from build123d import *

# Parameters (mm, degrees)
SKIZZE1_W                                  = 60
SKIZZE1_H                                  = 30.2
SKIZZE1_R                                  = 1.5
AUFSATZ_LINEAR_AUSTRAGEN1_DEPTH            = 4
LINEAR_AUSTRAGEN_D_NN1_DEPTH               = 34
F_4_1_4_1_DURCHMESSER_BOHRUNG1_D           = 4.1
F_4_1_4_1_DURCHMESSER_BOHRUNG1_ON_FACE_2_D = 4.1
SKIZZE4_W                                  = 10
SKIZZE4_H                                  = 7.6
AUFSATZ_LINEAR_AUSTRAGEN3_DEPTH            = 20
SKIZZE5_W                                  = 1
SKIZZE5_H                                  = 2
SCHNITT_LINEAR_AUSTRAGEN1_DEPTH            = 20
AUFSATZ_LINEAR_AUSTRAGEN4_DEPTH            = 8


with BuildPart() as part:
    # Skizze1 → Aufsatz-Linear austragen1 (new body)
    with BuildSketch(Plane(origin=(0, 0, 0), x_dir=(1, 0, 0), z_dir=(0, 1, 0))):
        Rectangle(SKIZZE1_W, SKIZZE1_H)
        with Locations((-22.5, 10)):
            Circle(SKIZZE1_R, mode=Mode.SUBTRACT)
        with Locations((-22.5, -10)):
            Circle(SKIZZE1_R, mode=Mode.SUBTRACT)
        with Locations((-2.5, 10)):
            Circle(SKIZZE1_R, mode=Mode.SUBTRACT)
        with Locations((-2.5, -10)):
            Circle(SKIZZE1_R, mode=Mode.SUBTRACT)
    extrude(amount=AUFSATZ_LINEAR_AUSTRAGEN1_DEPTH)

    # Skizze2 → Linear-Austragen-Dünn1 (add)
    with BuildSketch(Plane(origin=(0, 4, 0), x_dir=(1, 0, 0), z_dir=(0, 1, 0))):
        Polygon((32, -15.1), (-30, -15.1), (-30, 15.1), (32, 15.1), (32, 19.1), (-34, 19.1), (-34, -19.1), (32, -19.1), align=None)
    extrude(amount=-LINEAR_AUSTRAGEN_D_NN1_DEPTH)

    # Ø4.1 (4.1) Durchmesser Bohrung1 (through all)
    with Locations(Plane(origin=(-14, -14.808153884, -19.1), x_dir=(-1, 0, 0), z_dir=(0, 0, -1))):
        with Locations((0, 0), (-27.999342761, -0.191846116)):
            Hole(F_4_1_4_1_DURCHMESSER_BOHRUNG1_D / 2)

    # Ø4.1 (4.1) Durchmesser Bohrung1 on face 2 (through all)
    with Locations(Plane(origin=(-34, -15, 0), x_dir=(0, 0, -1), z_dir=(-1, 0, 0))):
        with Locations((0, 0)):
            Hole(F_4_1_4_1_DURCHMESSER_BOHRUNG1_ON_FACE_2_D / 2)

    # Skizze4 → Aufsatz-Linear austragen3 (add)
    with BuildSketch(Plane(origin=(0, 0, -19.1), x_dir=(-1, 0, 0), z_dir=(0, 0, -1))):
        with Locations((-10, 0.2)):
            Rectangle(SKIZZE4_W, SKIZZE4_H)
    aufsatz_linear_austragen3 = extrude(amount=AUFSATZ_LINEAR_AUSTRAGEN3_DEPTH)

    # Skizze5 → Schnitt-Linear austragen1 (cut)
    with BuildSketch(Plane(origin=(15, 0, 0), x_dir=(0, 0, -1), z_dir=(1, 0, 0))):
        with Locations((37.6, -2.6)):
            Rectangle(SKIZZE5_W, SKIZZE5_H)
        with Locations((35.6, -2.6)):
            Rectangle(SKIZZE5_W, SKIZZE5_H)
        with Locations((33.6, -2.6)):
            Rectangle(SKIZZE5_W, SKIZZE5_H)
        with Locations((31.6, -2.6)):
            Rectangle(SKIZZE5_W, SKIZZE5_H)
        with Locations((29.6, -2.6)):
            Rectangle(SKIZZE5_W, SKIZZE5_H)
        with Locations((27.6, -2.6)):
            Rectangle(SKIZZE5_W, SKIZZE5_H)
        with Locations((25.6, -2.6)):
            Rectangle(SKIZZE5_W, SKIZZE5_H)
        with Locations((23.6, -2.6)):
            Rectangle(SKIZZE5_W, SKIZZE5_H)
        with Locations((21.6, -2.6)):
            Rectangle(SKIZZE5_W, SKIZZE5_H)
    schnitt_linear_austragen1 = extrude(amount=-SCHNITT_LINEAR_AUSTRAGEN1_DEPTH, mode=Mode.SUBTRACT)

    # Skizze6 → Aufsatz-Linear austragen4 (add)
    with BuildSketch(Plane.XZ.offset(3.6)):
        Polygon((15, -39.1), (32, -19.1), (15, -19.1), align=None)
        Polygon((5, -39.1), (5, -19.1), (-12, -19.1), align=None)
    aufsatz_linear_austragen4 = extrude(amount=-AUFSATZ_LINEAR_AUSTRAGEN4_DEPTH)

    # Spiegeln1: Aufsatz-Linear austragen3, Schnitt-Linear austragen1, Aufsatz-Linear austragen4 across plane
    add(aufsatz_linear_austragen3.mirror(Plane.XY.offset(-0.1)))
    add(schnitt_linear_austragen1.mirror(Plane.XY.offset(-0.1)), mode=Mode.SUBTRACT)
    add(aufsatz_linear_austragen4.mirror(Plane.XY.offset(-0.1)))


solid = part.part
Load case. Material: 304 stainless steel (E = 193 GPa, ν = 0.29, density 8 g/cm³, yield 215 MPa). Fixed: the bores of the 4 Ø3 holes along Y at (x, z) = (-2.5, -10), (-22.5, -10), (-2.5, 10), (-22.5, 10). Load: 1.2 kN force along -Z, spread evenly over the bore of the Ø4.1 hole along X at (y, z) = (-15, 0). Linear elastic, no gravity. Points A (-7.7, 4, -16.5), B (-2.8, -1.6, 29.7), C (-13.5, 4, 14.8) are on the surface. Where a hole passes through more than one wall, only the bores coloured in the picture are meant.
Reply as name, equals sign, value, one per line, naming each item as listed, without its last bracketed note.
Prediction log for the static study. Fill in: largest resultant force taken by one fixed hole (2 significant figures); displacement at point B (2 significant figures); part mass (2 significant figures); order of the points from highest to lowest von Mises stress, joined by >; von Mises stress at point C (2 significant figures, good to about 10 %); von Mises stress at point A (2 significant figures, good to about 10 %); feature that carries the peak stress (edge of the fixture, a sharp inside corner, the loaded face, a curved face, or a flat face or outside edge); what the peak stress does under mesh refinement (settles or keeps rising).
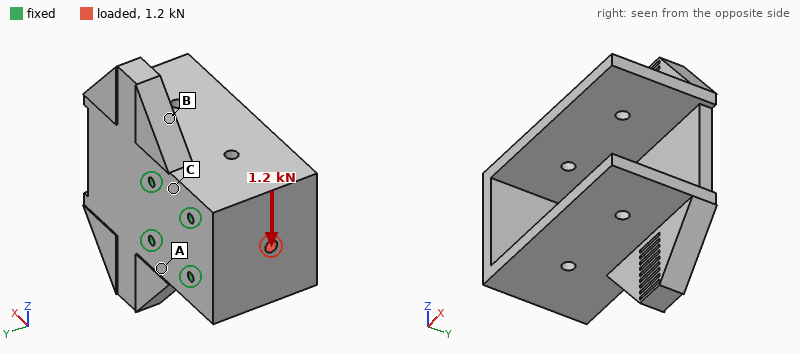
largest resultant force taken by one fixed hole = 1.0 kN
displacement at point B = 2.8 µm
part mass = 300 g
order of the points from highest to lowest von Mises stress, joined by > = C > A > B
von Mises stress at point C = 16 MPa
von Mises stress at point A = 8.5 MPa
feature that carries the peak stress = edge of the fixture
what the peak stress does under mesh refinement = keeps rising
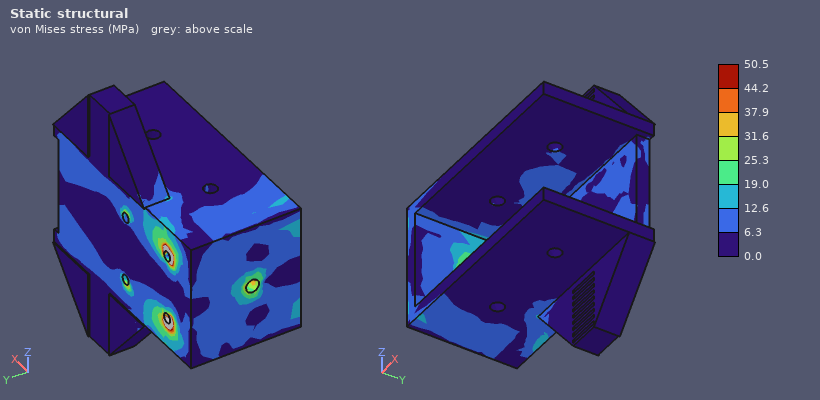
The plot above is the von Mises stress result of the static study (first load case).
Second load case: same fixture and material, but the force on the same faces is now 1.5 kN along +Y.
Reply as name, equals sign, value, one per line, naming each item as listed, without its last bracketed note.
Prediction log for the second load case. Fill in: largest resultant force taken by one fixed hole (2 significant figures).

largest resultant force taken by one fixed hole = 970 N
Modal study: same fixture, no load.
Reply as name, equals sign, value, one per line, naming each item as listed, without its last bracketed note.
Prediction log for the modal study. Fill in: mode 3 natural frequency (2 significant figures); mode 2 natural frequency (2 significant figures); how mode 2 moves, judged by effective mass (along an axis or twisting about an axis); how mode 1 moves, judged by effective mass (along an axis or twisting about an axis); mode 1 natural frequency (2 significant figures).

mode 3 natural frequency = 3900 Hz
mode 2 natural frequency = 2500 Hz
how mode 2 moves, judged by effective mass = along Z
how mode 1 moves, judged by effective mass = along Y
mode 1 natural frequency = 2400 Hz
